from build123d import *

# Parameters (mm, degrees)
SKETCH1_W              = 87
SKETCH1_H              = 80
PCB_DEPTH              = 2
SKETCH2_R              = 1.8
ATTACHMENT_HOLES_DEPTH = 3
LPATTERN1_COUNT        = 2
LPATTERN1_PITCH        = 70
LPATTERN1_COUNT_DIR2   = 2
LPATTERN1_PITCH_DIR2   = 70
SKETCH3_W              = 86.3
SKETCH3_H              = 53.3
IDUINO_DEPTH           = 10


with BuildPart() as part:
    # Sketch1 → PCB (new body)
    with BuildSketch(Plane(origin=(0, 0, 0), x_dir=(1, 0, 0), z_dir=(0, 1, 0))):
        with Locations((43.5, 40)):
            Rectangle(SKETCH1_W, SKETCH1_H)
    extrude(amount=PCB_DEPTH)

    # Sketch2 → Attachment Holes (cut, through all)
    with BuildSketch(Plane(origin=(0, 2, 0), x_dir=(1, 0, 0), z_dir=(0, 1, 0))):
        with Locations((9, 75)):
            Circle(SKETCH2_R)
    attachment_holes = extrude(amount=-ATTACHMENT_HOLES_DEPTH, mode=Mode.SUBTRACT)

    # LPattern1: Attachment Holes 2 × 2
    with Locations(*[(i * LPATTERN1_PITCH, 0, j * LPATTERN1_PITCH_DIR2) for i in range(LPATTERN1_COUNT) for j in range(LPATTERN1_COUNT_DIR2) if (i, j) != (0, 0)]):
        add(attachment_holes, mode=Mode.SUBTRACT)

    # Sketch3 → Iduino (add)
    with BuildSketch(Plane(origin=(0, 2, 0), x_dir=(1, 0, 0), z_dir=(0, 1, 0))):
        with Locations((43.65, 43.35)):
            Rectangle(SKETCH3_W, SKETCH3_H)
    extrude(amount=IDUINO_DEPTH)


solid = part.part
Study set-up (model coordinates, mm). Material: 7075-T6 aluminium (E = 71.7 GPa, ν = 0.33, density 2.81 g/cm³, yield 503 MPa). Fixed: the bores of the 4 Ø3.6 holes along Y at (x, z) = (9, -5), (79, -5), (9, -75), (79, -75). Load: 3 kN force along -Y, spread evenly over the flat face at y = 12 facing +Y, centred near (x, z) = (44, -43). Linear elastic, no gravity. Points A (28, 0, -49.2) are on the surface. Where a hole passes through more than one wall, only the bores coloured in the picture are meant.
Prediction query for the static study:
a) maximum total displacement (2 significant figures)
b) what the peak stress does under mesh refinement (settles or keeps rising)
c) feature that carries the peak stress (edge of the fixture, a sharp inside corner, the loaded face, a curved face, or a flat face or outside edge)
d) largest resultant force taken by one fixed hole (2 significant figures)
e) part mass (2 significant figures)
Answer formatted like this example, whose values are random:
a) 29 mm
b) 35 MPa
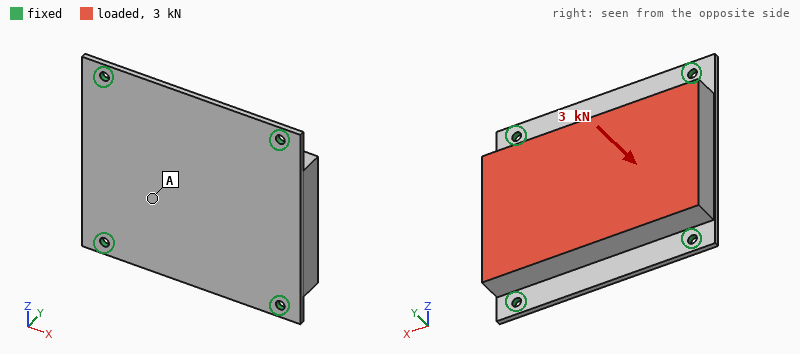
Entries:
a) 0.13 mm
b) keeps rising
c) edge of the fixture
d) 1.1 kN
e) 170 g
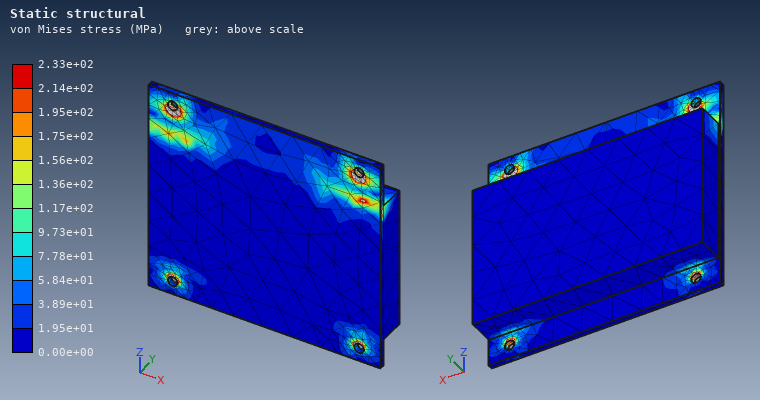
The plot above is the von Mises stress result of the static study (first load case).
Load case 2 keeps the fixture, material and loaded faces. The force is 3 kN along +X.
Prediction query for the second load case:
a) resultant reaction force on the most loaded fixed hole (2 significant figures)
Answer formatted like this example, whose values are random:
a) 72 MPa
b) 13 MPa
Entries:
a) 1.1 kN
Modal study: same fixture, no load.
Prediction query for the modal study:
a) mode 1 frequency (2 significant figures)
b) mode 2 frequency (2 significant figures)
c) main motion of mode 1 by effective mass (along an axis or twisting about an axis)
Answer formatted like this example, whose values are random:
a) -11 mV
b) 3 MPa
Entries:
a) 2200 Hz
b) 3900 Hz
c) along Y
